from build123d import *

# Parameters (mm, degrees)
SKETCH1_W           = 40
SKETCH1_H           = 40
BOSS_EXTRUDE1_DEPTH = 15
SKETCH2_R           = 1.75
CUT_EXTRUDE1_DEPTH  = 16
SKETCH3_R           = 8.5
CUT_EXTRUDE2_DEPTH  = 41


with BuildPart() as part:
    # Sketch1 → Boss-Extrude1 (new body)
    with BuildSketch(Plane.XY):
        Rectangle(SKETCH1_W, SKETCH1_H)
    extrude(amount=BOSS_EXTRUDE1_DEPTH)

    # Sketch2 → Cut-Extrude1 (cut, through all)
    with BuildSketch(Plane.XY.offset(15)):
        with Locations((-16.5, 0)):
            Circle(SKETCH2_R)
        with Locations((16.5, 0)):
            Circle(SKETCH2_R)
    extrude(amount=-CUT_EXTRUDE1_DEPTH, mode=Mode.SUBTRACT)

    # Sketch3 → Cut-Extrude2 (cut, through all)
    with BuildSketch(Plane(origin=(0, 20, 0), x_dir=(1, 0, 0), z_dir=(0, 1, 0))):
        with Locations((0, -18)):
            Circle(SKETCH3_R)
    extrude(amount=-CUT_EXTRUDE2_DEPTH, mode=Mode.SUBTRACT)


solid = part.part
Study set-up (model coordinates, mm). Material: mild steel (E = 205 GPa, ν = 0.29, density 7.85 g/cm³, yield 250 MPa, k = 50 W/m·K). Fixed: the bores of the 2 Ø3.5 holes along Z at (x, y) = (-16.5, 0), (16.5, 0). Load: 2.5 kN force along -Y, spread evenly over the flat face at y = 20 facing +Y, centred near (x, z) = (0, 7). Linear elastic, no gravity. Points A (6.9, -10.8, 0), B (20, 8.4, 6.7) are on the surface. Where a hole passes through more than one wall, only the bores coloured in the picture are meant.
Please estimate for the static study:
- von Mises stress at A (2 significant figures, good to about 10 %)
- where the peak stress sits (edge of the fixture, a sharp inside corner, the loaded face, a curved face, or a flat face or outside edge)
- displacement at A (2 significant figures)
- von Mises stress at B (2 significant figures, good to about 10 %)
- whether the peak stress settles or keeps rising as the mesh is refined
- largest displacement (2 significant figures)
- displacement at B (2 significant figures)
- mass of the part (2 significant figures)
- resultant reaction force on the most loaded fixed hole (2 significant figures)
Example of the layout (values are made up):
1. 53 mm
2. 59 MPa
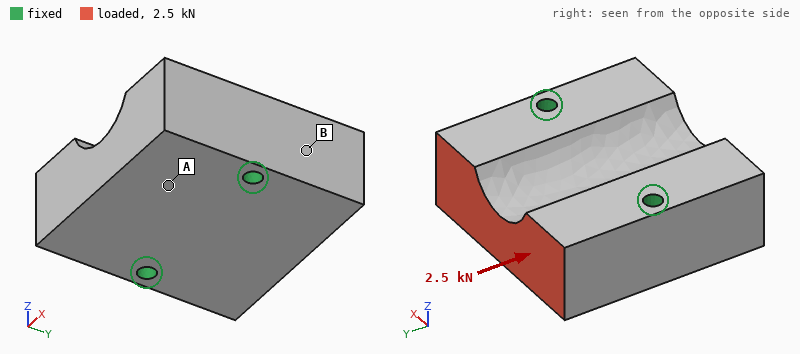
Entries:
1. 2.2 MPa
2. edge of the fixture
3. 0.30 µm
4. 6.0 MPa
5. keeps rising
6. 0.79 µm
7. 0.24 µm
8. 170 g
9. 1.3 kN
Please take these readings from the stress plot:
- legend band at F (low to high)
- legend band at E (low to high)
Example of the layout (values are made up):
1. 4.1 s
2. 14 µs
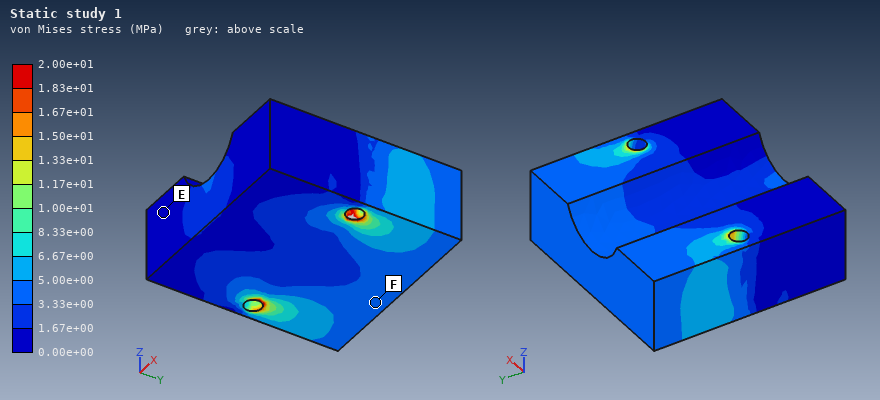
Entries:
1. 3.33e+00 to 5.00e+00 MPa
2. 0.00e+00 to 1.67e+00 MPa
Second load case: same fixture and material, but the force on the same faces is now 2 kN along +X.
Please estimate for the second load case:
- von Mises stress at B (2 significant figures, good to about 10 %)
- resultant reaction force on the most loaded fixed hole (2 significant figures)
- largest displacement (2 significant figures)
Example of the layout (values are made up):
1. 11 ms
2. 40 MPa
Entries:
1. 8.6 MPa
2. 1.5 kN
3. 2.2 µm
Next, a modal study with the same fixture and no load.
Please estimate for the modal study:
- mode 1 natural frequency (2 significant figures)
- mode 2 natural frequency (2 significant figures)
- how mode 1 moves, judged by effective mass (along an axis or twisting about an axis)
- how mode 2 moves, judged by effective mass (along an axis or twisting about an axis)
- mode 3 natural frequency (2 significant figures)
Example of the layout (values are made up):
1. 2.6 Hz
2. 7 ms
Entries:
1. 17 kHz
2. 20 kHz
3. twisting about X
4. along Z
5. 25 kHz
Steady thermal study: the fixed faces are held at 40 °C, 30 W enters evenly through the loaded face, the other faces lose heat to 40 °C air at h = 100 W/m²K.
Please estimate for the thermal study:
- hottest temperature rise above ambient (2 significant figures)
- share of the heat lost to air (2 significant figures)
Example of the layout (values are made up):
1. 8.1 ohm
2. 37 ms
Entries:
1. 24 K
2. 12 %
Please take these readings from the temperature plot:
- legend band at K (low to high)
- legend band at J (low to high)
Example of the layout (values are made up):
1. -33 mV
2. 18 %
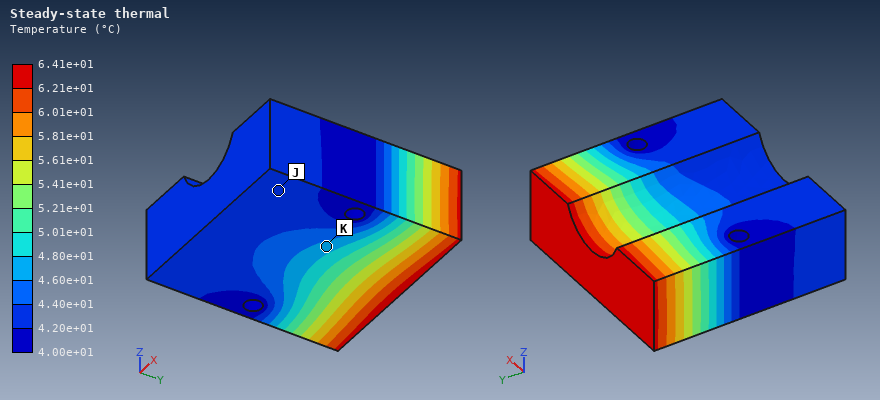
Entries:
1. 4.60e+01 to 4.80e+01 °C
2. 4.20e+01 to 4.40e+01 °C
